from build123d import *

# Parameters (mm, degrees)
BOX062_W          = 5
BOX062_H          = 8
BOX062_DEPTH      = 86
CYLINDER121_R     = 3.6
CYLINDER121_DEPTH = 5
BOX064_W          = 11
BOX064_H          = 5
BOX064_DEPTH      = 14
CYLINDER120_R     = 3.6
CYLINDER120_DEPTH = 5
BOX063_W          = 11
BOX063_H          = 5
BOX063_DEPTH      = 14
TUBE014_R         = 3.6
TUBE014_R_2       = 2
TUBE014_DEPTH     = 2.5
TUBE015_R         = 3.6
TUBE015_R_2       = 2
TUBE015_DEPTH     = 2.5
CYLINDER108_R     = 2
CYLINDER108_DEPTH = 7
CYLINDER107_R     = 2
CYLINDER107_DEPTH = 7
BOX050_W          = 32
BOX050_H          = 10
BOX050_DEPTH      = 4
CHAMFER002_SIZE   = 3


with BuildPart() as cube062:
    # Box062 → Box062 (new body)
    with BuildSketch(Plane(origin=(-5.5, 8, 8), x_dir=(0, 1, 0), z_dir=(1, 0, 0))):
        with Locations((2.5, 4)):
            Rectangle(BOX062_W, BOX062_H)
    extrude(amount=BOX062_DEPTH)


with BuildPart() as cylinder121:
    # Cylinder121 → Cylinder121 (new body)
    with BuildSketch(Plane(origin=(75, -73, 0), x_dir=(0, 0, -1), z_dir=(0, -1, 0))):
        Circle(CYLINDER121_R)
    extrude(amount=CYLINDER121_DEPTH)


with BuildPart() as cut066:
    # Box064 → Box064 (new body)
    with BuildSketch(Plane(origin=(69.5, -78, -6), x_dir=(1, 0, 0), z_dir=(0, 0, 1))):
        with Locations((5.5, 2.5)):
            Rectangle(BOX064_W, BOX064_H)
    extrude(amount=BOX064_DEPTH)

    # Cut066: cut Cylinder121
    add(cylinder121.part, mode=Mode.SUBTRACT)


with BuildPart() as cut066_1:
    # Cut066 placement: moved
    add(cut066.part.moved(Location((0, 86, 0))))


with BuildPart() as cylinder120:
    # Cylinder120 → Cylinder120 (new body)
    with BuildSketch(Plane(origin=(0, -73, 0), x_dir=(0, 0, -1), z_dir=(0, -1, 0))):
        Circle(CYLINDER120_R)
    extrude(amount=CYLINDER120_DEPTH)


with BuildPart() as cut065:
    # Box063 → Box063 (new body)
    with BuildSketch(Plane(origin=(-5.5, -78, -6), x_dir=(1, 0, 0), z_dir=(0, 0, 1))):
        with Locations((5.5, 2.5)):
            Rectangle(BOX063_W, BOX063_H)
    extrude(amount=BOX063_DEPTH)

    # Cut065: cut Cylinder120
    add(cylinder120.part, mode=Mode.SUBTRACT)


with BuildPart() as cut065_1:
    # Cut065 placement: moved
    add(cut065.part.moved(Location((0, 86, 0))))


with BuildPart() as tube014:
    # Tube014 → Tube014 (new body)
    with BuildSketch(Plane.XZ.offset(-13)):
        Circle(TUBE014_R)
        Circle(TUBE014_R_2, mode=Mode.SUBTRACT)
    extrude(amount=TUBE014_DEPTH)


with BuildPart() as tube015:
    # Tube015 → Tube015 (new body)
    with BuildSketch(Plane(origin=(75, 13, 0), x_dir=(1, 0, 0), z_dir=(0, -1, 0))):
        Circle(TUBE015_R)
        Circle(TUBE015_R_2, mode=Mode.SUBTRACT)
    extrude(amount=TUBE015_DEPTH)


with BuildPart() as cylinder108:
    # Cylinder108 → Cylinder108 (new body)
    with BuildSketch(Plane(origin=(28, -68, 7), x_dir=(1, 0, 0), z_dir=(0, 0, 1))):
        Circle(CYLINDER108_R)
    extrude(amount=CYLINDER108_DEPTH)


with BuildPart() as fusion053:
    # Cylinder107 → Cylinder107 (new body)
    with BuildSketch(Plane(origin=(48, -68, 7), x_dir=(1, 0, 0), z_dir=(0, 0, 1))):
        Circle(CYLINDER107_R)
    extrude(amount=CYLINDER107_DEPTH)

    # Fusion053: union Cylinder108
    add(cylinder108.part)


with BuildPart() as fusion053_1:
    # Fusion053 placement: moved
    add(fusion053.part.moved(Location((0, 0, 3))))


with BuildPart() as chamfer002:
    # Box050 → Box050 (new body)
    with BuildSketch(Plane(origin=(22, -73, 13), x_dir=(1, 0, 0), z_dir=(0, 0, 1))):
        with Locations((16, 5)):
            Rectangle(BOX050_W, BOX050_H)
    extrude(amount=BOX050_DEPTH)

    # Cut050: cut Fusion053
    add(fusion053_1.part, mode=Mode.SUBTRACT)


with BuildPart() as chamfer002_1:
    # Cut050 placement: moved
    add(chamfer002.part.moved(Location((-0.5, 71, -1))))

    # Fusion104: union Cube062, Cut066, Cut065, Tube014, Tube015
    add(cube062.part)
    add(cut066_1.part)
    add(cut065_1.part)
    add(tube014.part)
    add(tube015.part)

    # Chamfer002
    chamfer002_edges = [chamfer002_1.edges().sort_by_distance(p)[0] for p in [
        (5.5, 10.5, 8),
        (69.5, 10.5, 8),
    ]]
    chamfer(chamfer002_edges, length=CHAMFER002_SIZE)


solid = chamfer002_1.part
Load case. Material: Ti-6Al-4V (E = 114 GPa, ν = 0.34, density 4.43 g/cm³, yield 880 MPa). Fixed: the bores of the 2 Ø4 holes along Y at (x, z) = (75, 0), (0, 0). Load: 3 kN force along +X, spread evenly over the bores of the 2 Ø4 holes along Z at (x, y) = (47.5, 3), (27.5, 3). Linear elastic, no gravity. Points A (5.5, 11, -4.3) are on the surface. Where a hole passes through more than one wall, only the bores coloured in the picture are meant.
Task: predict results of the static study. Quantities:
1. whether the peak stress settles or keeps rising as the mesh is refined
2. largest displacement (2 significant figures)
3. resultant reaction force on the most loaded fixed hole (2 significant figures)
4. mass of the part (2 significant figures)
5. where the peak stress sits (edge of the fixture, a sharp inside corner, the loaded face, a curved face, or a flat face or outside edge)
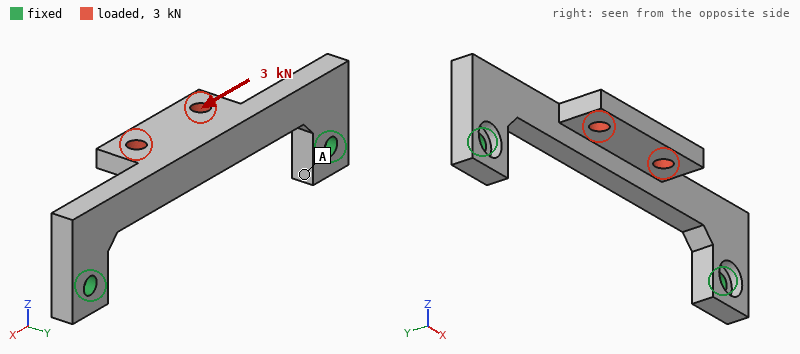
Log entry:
keeps rising
0.11 mm
1.6 kN
26 g
edge of the fixture
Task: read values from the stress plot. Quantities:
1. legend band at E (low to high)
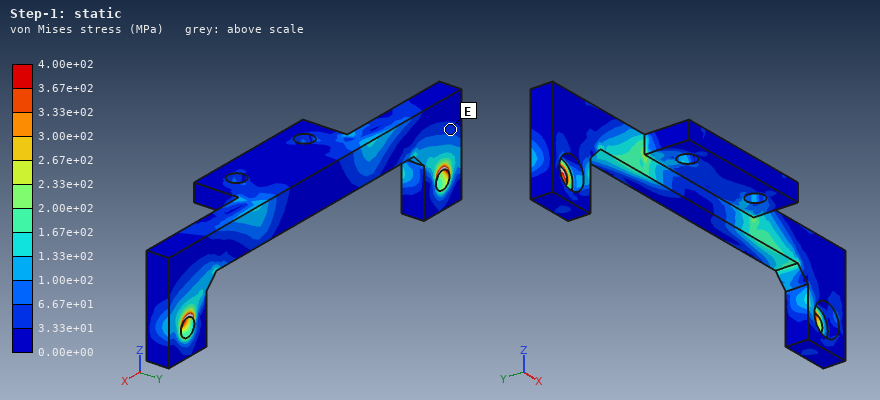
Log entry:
3.33e+01 to 6.67e+01 MPa
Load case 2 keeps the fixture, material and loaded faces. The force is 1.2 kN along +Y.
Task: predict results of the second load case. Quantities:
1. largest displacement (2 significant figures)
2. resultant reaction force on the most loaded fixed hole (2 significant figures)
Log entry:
0.32 mm
610 N
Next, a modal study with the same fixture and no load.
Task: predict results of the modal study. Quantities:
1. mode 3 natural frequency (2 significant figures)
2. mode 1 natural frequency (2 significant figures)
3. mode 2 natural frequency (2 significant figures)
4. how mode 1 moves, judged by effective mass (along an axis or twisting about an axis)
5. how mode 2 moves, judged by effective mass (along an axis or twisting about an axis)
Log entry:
6800 Hz
2800 Hz
5300 Hz
along Y
along Z
